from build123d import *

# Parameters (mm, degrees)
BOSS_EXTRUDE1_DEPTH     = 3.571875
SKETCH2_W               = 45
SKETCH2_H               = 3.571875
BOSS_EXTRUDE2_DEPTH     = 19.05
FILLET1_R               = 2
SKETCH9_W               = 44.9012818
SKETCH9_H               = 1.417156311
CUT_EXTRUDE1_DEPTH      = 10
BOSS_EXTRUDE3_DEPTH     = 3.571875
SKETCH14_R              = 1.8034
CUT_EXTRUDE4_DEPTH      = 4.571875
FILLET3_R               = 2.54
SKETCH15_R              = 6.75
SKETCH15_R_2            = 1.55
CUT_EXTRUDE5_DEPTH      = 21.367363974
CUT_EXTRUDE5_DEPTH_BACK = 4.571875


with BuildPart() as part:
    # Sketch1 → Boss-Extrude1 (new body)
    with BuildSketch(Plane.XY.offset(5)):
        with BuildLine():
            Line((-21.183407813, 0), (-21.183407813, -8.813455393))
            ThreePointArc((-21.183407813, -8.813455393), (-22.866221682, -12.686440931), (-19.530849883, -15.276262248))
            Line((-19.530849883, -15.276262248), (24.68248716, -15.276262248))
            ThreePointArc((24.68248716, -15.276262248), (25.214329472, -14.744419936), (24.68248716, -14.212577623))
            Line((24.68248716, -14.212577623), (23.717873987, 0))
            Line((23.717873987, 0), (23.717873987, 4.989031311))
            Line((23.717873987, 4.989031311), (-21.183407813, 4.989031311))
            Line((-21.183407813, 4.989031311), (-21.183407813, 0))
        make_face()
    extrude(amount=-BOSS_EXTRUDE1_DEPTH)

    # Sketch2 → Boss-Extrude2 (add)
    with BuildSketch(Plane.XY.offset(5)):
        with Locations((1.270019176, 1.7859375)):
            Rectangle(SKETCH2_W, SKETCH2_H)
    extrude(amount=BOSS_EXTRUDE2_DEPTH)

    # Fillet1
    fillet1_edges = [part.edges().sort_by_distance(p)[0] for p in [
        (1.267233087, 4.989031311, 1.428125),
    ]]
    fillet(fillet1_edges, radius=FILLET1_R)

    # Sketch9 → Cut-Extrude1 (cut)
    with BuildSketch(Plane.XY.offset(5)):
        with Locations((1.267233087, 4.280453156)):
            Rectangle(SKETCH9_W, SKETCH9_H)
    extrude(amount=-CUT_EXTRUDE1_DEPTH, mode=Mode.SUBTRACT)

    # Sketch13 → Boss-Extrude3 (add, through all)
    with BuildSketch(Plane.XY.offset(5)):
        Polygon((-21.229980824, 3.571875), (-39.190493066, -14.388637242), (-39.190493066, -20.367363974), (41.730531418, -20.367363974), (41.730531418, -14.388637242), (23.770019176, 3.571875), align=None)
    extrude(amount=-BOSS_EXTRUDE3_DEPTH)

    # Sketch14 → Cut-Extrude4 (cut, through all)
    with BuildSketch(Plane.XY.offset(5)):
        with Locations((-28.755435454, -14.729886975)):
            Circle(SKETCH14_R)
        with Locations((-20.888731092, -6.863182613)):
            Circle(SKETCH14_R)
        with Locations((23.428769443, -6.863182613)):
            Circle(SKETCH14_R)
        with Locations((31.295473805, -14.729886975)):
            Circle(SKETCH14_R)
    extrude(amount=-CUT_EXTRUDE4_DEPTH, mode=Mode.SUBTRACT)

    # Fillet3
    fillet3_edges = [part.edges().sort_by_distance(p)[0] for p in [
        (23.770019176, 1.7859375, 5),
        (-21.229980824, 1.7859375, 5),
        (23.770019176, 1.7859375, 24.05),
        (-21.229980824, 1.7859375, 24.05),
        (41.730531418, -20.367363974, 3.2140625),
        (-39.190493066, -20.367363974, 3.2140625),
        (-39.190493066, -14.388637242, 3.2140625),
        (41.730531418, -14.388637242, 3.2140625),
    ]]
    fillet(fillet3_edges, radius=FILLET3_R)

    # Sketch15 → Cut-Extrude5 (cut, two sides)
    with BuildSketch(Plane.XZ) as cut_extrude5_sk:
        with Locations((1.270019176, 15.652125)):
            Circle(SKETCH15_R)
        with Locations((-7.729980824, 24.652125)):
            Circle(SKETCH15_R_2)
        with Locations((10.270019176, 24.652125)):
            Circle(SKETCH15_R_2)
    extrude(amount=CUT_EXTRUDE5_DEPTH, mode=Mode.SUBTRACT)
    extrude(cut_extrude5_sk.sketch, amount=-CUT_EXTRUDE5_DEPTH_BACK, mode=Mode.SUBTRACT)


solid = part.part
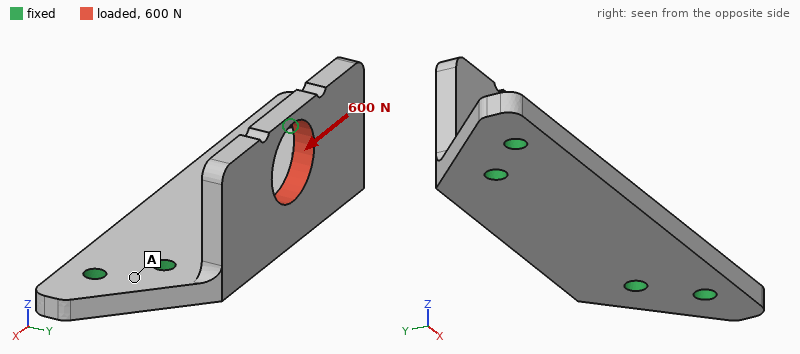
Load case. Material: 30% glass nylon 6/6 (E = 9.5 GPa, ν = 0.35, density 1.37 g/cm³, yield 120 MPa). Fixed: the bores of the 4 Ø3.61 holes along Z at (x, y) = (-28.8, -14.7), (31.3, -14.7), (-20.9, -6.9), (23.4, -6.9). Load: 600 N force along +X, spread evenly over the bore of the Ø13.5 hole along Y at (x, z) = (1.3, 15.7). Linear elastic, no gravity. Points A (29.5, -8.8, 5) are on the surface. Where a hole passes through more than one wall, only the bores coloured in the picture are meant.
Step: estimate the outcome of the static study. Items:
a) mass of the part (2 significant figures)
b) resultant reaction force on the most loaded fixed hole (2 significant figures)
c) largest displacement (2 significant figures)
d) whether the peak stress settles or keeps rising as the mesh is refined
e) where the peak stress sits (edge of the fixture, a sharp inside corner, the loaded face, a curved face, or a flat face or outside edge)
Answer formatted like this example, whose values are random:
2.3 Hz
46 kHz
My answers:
11 g
320 N
0.14 mm
keeps rising
edge of the fixture
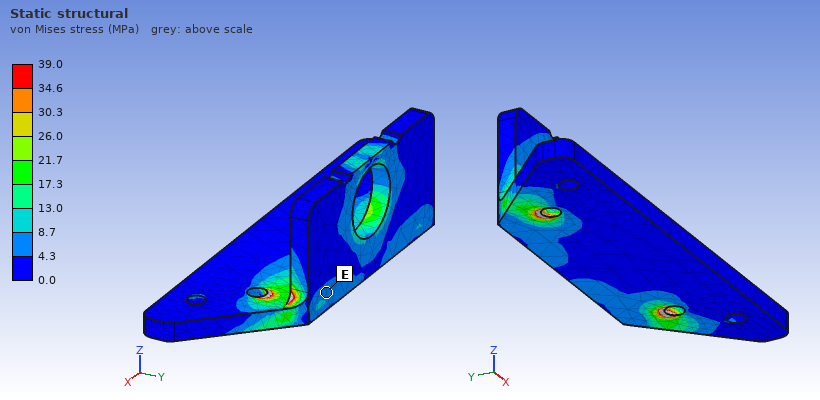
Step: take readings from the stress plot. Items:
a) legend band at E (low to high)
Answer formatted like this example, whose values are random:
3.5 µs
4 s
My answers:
4.3 to 8.7 MPa
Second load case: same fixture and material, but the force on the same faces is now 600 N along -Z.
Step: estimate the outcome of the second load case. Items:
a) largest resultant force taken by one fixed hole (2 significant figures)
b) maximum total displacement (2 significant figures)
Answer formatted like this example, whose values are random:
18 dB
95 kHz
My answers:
390 N
0.39 mm
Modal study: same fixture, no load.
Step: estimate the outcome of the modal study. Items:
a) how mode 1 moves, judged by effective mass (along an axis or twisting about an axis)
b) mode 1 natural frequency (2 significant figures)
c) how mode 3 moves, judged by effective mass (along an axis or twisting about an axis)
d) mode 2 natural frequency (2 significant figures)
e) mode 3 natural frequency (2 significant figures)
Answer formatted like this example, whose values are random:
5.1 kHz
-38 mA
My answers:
along Y
2200 Hz
along Z
3700 Hz
4900 Hz
